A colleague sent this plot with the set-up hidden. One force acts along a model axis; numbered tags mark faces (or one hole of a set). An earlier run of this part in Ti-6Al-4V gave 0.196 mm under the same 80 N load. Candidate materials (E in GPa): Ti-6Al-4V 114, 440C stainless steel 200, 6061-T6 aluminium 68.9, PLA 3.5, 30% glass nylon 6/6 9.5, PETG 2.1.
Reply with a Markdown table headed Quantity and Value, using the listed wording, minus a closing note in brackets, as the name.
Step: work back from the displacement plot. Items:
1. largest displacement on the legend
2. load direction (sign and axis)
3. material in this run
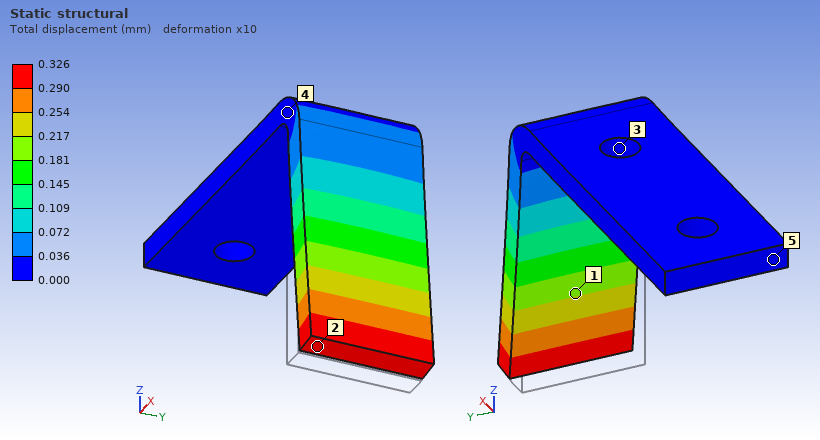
| Quantity | Value |
|---|---|
| largest displacement on the legend | 0.326 mm |
| load direction | +X |
| material in this run | 6061-T6 aluminium |
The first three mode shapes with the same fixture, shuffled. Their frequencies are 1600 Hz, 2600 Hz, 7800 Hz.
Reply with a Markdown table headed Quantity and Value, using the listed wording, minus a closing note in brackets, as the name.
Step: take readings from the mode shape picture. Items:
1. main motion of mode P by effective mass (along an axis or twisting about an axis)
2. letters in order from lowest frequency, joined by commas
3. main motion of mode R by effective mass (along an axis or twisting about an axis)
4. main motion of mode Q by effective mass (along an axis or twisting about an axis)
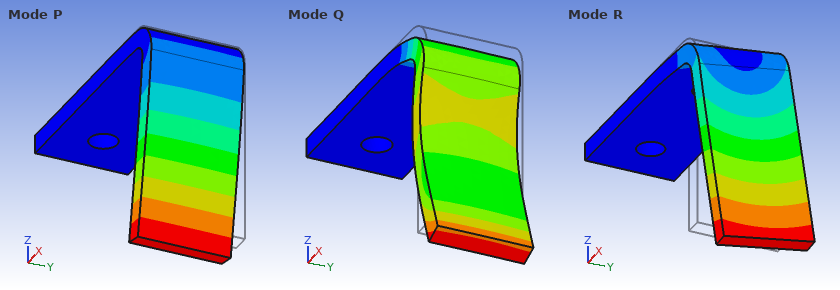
| Quantity | Value |
|---|---|
| main motion of mode P by effective mass | along X |
| letters in order from lowest frequency, joined by commas | P, R, Q |
| main motion of mode R by effective mass | along Y |
| main motion of mode Q by effective mass | along Z |
